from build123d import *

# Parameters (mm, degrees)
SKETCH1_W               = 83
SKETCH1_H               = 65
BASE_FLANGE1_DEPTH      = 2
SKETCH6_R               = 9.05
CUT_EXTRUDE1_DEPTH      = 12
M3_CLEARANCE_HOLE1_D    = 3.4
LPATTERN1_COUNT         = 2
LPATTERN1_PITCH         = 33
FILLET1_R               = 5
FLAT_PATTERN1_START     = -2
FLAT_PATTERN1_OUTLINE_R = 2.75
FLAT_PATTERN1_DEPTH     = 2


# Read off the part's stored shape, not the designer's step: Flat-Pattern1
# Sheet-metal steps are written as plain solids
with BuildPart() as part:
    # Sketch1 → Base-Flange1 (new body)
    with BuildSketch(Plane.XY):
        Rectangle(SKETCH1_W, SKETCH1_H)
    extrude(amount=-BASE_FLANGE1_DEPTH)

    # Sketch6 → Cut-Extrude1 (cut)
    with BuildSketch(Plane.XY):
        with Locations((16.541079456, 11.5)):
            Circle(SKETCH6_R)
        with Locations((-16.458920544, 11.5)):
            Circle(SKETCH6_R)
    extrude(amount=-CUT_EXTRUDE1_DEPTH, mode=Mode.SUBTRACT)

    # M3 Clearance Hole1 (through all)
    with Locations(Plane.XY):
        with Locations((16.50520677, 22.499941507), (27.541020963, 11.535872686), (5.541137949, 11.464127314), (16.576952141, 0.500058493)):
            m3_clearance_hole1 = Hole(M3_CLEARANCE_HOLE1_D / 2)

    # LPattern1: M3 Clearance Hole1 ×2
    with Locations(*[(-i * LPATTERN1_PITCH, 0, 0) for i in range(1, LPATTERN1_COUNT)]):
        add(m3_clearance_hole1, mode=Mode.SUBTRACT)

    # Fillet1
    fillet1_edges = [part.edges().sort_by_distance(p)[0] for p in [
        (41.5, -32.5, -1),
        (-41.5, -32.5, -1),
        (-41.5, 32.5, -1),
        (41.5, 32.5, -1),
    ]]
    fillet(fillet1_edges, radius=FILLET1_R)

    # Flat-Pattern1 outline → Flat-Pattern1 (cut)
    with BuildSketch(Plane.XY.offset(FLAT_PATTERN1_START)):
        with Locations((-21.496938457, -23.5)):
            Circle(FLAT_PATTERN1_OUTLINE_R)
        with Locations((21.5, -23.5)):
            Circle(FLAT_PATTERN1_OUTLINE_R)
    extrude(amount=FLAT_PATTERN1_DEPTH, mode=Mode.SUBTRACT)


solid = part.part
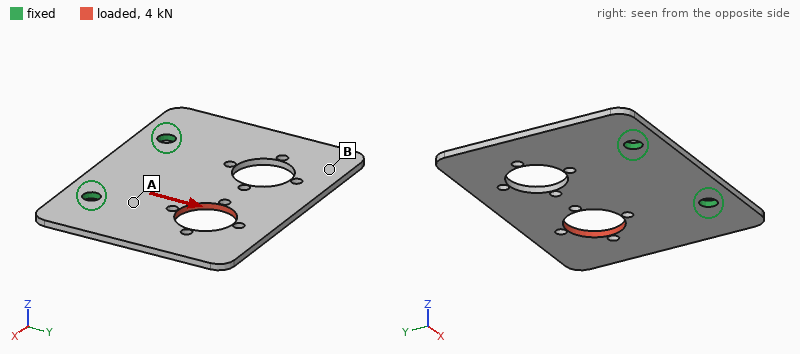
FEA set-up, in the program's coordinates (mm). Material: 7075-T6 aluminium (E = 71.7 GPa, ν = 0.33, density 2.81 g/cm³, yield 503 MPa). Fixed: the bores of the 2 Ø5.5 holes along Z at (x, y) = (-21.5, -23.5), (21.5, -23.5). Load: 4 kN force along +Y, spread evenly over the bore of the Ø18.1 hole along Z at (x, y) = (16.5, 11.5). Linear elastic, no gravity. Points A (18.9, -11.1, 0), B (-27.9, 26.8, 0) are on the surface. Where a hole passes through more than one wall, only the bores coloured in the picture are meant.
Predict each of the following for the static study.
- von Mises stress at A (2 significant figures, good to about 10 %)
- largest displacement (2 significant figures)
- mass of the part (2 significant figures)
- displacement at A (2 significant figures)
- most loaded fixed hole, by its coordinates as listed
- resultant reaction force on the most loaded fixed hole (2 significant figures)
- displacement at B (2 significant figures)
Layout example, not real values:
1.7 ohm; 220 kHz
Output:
69 MPa; 72 µm; 27 g; 14 µm; (21.5, -23.5); 3.4 kN; 27 µm
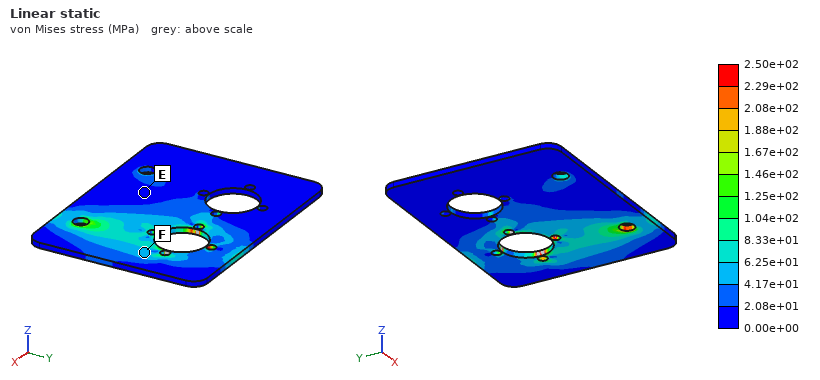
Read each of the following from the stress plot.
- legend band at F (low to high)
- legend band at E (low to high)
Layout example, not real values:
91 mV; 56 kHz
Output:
4.17e+01 to 6.25e+01 MPa; 0.00e+00 to 2.08e+01 MPa
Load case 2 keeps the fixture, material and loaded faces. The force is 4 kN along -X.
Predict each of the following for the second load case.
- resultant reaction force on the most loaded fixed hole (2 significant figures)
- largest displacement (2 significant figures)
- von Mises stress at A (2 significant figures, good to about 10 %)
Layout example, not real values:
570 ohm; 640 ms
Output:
3.6 kN; 0.15 mm; 81 MPa
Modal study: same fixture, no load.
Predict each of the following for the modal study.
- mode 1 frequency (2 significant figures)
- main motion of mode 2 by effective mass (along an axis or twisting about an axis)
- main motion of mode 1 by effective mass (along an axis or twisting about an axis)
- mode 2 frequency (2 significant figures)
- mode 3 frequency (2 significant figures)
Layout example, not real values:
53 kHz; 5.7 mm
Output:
530 Hz; twisting about Y; along Z; 890 Hz; 1800 Hz
